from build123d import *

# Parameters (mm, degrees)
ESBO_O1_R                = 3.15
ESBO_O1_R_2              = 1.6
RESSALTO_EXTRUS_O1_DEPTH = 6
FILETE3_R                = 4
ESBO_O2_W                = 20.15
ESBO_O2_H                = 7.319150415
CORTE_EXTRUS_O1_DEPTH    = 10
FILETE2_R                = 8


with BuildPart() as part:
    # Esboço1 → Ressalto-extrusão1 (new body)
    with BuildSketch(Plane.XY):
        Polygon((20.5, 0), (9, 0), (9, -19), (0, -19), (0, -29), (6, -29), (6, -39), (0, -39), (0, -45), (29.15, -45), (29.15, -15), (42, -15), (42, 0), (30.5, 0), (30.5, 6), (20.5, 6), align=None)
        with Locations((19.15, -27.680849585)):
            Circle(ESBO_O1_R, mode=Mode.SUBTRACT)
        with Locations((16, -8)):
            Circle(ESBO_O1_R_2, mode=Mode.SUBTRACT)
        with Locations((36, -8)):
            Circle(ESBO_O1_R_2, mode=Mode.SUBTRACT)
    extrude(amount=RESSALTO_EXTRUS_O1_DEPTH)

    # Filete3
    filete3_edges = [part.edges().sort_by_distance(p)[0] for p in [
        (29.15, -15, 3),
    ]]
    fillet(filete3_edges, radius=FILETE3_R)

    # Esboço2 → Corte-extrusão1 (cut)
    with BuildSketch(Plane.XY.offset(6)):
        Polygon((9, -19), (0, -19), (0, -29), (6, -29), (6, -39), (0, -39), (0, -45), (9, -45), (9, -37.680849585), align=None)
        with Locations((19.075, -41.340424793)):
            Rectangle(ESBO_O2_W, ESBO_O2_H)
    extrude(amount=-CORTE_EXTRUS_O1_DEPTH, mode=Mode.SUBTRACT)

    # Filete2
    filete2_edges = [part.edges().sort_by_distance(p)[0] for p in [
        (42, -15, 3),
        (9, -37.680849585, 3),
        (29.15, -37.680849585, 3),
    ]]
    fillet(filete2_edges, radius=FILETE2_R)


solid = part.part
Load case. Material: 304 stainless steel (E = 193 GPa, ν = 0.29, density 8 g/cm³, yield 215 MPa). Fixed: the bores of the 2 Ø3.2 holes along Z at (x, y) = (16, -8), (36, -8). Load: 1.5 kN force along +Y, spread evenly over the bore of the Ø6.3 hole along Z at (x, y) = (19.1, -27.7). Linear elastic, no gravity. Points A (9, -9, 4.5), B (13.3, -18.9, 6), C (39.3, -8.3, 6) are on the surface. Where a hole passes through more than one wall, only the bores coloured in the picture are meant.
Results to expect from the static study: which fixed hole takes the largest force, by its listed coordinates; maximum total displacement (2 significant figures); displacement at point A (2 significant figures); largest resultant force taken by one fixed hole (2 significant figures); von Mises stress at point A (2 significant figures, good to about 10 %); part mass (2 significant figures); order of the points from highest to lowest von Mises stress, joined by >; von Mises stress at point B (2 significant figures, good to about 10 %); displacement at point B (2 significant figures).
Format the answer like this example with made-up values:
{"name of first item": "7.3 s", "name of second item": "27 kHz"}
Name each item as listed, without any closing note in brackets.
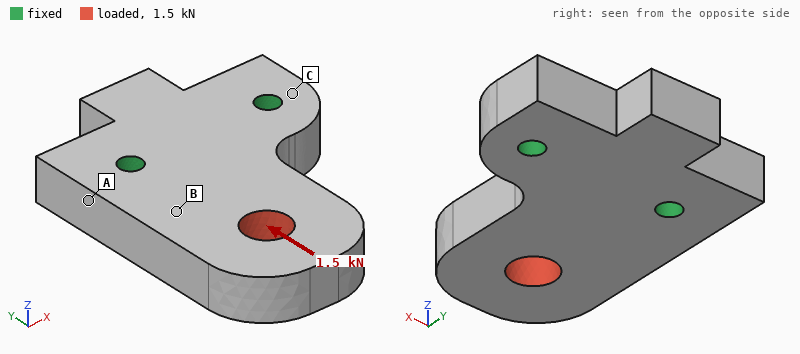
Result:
{"which fixed hole takes the largest force, by its listed coordinates": "(16, -8)", "maximum total displacement": "2.2 µm", "displacement at point A": "0.58 µm", "largest resultant force taken by one fixed hole": "1.2 kN", "von Mises stress at point A": "7.1 MPa", "part mass": "44 g", "order of the points from highest to lowest von Mises stress, joined by >": "B > A > C", "von Mises stress at point B": "14 MPa", "displacement at point B": "1.0 µm"}
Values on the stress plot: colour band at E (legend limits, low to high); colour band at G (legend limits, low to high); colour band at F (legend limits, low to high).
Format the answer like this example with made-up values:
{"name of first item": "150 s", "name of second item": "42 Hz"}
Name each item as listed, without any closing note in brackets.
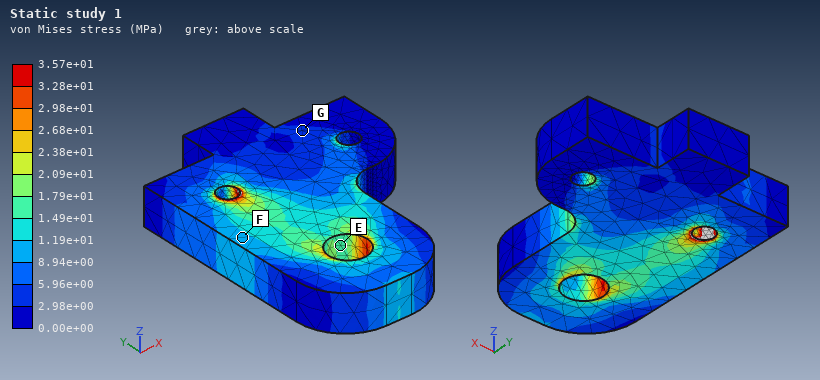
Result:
{"colour band at E": "1.49e+01 to 1.79e+01 MPa", "colour band at G": "2.98e+00 to 5.96e+00 MPa", "colour band at F": "8.94e+00 to 1.19e+01 MPa"}
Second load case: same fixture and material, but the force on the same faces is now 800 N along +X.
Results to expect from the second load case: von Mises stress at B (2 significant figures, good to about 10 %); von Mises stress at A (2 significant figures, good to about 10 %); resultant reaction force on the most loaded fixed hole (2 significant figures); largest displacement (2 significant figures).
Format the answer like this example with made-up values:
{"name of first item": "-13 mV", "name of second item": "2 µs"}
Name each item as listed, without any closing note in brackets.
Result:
{"von Mises stress at B": "10 MPa", "von Mises stress at A": "15 MPa", "resultant reaction force on the most loaded fixed hole": "840 N", "largest displacement": "6.9 µm"}
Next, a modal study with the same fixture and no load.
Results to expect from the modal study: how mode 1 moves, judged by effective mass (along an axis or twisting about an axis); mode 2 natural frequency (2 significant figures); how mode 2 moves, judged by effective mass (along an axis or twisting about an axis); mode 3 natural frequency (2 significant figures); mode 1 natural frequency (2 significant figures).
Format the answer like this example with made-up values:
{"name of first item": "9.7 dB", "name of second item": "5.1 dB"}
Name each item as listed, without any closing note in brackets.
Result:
{"how mode 1 moves, judged by effective mass": "along Z", "mode 2 natural frequency": "15 kHz", "how mode 2 moves, judged by effective mass": "along X", "mode 3 natural frequency": "17 kHz", "mode 1 natural frequency": "5800 Hz"}
